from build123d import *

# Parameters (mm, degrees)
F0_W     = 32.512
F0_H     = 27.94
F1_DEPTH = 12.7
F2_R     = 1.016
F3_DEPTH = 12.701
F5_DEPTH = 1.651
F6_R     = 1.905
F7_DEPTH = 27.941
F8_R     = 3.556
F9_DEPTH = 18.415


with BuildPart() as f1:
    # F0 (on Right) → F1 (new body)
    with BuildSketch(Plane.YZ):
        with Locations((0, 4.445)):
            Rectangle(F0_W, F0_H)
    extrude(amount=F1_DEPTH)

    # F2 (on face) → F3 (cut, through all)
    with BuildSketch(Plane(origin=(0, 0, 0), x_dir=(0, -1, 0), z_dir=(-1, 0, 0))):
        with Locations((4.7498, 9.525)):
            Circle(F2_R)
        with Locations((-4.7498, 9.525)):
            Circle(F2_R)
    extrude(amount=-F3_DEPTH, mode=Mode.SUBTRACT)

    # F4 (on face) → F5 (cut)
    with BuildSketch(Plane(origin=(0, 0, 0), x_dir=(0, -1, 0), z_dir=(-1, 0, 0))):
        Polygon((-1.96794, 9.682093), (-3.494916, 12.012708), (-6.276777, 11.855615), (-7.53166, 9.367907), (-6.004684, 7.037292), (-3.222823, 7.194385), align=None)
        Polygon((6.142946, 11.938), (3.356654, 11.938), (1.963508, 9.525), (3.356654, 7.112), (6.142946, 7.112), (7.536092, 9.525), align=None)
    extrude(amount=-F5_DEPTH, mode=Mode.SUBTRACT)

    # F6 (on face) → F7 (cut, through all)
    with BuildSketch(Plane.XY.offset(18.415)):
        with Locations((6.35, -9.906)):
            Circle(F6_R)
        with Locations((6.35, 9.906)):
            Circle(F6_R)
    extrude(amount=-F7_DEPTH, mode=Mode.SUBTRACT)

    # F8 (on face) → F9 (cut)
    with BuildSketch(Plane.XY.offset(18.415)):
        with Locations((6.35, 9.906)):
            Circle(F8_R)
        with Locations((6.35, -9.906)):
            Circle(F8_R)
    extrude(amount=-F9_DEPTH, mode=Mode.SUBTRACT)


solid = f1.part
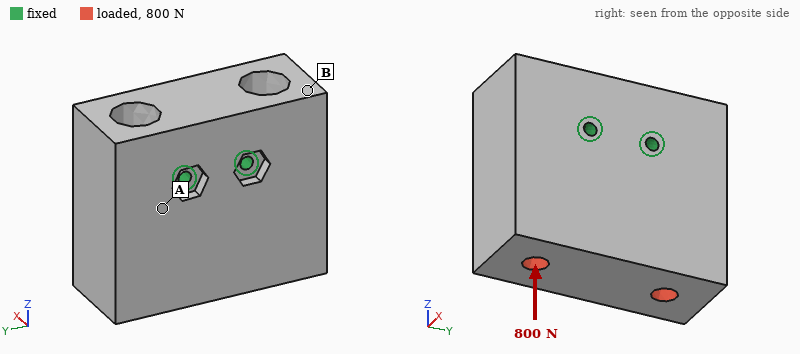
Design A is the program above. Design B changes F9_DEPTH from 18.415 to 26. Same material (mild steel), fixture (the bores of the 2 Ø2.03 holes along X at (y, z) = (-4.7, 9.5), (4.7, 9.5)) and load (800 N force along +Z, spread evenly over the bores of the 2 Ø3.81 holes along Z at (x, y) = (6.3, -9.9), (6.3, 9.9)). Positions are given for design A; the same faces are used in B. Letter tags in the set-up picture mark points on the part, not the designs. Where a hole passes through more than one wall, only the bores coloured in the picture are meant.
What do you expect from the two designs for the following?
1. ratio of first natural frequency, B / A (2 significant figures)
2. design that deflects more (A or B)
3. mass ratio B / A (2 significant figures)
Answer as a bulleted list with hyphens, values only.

- 1.0
- B
- 0.96
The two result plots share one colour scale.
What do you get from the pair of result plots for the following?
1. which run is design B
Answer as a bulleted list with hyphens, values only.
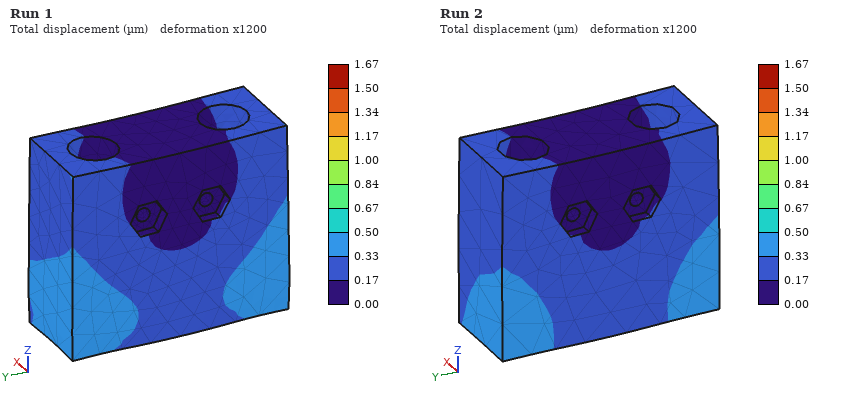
- Run 1
